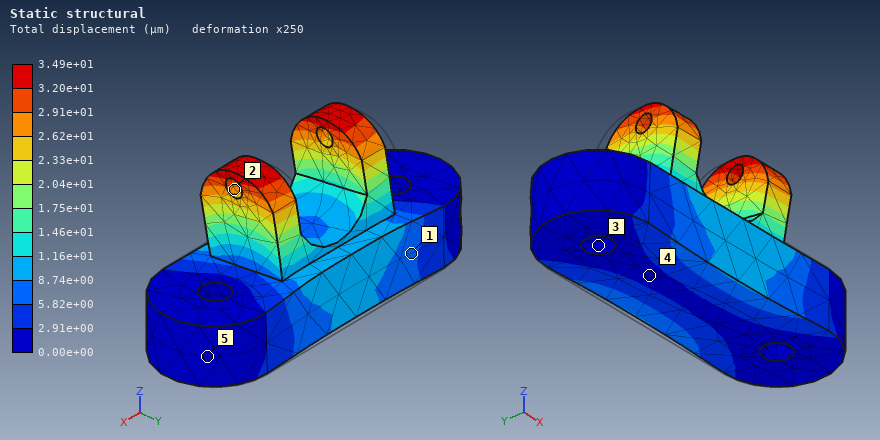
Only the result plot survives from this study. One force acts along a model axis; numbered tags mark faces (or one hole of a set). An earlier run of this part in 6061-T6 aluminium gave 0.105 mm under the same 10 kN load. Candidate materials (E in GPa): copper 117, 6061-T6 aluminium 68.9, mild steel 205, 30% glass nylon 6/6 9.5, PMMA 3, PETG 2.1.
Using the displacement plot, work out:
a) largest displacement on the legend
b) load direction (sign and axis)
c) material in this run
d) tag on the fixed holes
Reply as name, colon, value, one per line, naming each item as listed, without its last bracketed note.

largest displacement on the legend: 3.49e+01 µm
load direction: -Y
material in this run: mild steel
tag on the fixed holes: 3
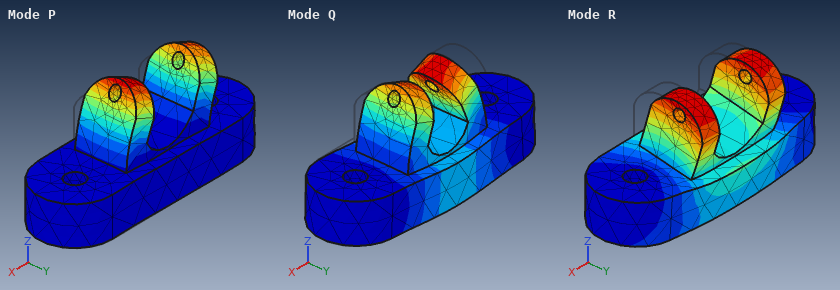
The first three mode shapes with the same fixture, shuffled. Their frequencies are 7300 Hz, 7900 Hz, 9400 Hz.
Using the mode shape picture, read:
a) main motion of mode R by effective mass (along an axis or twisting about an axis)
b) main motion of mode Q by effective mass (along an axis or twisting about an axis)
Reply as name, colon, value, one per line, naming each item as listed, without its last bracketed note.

main motion of mode R by effective mass: along Y
main motion of mode Q by effective mass: along Z
